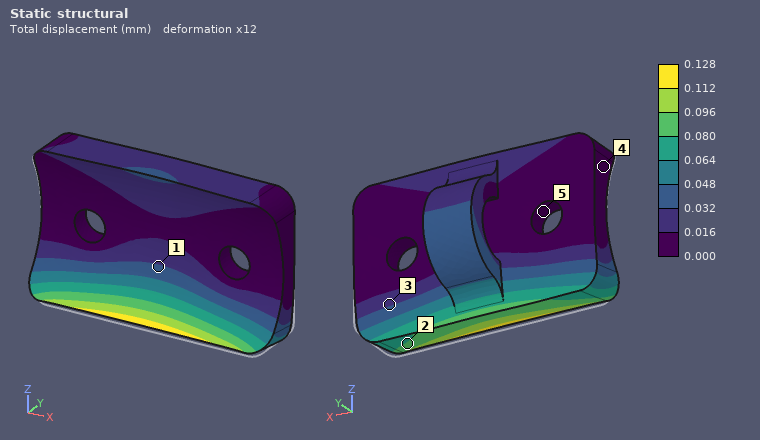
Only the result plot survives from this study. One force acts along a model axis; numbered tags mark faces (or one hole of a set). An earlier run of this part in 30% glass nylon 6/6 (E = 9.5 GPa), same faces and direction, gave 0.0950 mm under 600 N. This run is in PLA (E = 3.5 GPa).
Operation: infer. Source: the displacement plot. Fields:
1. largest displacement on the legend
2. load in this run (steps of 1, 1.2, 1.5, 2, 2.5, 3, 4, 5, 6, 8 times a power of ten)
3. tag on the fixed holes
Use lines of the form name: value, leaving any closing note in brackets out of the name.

largest displacement on the legend: 0.128 mm
load in this run: 300 N
tag on the fixed holes: 5
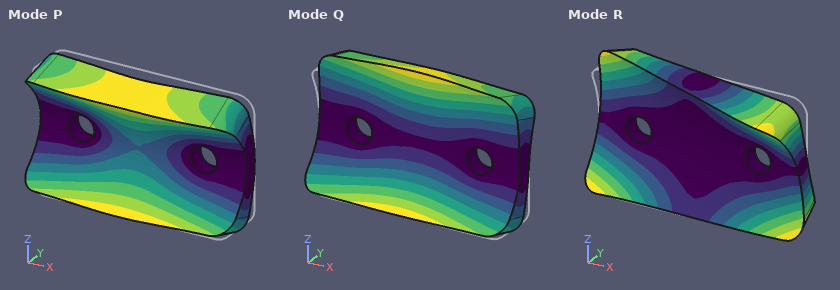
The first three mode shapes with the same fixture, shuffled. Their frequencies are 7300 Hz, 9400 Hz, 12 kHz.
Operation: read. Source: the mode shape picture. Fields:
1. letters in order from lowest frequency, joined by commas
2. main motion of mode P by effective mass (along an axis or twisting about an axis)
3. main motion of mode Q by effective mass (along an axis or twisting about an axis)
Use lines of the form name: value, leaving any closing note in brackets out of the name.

letters in order from lowest frequency, joined by commas: Q, P, R
main motion of mode P by effective mass: along Y
main motion of mode Q by effective mass: twisting about X
